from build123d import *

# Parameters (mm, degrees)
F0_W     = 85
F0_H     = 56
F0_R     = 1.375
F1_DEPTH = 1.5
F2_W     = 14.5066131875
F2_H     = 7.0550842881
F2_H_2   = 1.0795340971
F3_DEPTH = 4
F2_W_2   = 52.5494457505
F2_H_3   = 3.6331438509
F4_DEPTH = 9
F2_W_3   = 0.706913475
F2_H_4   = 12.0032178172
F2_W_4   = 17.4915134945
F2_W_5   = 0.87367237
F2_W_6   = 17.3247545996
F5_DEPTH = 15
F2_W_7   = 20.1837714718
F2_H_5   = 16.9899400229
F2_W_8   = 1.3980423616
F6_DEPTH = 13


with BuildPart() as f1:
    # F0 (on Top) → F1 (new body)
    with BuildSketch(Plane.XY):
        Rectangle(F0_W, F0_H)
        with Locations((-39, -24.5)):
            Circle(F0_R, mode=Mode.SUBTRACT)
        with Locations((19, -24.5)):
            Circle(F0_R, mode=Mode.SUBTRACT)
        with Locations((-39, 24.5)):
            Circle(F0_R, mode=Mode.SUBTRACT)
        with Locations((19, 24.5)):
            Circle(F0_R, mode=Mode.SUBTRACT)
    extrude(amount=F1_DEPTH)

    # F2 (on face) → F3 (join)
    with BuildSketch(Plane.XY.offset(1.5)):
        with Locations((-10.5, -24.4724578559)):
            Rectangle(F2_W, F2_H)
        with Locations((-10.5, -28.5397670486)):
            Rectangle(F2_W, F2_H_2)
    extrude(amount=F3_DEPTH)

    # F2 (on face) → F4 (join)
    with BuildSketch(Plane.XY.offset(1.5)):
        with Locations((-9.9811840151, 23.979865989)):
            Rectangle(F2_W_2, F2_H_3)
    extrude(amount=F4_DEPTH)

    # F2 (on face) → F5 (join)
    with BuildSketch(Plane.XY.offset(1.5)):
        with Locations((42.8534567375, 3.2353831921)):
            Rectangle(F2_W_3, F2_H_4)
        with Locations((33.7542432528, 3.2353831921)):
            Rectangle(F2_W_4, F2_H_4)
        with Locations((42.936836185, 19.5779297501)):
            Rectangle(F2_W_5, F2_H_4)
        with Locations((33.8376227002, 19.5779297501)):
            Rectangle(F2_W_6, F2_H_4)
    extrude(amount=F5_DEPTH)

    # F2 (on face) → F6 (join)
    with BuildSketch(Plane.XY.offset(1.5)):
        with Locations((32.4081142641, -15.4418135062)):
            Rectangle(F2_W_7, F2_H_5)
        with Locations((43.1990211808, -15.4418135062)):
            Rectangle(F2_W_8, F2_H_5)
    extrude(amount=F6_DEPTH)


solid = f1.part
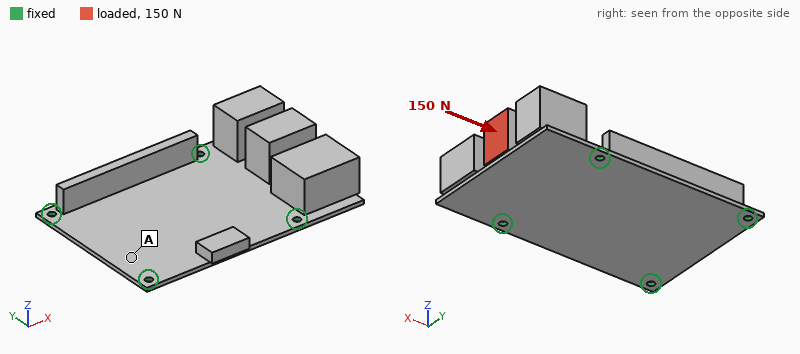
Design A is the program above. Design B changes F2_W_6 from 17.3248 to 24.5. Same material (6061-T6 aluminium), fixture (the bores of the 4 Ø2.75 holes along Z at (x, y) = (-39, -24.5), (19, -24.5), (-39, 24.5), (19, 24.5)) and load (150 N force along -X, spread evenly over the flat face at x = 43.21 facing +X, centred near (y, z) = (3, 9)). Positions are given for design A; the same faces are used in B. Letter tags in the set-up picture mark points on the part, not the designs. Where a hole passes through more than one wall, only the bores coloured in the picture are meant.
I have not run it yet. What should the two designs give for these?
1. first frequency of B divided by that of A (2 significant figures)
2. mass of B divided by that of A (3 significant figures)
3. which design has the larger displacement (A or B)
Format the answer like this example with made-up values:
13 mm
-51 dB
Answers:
1.0
1.06
A
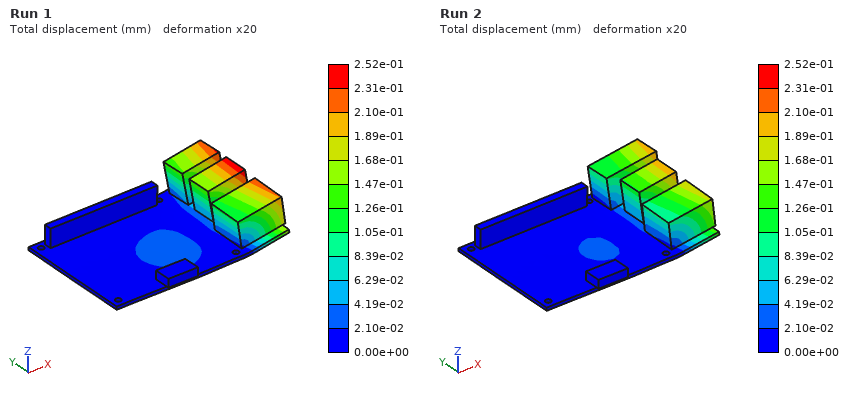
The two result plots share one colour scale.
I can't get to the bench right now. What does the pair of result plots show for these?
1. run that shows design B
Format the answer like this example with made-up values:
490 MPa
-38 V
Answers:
Run 2
